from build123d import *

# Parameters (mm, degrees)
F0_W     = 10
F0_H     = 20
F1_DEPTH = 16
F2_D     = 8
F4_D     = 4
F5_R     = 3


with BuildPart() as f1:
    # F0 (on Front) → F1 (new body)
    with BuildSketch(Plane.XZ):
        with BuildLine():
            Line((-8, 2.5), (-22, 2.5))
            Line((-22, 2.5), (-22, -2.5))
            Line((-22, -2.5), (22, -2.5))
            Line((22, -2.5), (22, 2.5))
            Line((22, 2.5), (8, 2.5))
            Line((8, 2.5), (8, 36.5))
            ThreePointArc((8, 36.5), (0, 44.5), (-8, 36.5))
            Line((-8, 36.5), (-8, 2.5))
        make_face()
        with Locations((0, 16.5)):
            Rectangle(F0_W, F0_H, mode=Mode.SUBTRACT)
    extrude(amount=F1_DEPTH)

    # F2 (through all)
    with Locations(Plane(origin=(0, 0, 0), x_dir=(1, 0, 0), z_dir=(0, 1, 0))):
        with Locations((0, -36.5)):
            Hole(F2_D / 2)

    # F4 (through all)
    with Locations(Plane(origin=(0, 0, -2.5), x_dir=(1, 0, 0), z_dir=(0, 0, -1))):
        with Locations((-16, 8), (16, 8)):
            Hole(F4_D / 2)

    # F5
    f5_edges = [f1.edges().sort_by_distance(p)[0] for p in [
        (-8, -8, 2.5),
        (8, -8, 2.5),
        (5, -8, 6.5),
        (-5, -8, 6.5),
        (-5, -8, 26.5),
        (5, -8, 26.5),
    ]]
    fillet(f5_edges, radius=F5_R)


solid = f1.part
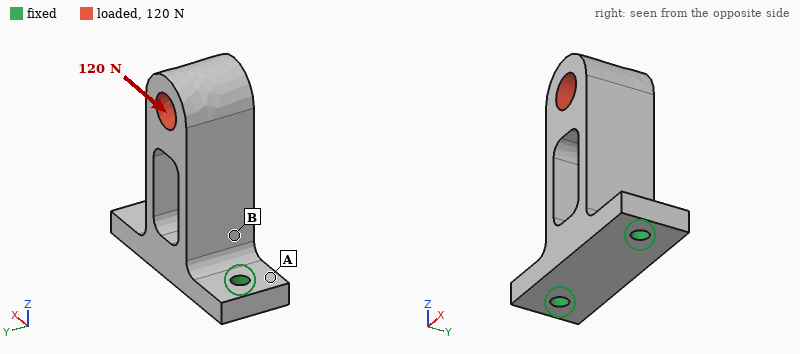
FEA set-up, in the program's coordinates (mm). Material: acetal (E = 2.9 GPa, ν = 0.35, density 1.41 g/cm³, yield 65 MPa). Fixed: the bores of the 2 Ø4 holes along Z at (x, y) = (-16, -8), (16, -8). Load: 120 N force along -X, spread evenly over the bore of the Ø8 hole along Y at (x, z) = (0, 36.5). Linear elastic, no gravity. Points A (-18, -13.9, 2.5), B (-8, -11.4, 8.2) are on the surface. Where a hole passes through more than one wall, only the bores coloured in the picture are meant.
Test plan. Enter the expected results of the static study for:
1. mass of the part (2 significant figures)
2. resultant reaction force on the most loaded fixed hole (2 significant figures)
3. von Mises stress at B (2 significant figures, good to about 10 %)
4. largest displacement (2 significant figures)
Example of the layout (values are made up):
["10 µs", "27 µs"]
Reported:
["14 g", "180 N", "20 MPa", "0.71 mm"]
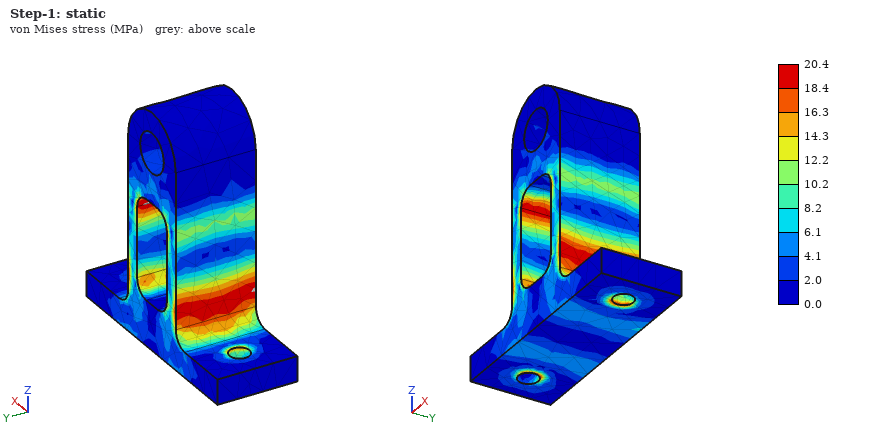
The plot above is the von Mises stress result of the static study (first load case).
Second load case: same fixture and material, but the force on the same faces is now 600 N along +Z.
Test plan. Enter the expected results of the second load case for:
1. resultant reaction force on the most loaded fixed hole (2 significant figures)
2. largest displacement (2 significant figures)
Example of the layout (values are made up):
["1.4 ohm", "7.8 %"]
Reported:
["330 N", "0.15 mm"]
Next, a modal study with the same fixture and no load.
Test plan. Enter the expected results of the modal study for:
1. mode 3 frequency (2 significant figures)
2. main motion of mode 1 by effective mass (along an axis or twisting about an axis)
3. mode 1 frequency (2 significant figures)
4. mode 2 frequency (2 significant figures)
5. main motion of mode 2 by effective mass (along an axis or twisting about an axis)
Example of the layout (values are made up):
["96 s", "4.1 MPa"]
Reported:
["2700 Hz", "along Y", "730 Hz", "950 Hz", "along X"]
